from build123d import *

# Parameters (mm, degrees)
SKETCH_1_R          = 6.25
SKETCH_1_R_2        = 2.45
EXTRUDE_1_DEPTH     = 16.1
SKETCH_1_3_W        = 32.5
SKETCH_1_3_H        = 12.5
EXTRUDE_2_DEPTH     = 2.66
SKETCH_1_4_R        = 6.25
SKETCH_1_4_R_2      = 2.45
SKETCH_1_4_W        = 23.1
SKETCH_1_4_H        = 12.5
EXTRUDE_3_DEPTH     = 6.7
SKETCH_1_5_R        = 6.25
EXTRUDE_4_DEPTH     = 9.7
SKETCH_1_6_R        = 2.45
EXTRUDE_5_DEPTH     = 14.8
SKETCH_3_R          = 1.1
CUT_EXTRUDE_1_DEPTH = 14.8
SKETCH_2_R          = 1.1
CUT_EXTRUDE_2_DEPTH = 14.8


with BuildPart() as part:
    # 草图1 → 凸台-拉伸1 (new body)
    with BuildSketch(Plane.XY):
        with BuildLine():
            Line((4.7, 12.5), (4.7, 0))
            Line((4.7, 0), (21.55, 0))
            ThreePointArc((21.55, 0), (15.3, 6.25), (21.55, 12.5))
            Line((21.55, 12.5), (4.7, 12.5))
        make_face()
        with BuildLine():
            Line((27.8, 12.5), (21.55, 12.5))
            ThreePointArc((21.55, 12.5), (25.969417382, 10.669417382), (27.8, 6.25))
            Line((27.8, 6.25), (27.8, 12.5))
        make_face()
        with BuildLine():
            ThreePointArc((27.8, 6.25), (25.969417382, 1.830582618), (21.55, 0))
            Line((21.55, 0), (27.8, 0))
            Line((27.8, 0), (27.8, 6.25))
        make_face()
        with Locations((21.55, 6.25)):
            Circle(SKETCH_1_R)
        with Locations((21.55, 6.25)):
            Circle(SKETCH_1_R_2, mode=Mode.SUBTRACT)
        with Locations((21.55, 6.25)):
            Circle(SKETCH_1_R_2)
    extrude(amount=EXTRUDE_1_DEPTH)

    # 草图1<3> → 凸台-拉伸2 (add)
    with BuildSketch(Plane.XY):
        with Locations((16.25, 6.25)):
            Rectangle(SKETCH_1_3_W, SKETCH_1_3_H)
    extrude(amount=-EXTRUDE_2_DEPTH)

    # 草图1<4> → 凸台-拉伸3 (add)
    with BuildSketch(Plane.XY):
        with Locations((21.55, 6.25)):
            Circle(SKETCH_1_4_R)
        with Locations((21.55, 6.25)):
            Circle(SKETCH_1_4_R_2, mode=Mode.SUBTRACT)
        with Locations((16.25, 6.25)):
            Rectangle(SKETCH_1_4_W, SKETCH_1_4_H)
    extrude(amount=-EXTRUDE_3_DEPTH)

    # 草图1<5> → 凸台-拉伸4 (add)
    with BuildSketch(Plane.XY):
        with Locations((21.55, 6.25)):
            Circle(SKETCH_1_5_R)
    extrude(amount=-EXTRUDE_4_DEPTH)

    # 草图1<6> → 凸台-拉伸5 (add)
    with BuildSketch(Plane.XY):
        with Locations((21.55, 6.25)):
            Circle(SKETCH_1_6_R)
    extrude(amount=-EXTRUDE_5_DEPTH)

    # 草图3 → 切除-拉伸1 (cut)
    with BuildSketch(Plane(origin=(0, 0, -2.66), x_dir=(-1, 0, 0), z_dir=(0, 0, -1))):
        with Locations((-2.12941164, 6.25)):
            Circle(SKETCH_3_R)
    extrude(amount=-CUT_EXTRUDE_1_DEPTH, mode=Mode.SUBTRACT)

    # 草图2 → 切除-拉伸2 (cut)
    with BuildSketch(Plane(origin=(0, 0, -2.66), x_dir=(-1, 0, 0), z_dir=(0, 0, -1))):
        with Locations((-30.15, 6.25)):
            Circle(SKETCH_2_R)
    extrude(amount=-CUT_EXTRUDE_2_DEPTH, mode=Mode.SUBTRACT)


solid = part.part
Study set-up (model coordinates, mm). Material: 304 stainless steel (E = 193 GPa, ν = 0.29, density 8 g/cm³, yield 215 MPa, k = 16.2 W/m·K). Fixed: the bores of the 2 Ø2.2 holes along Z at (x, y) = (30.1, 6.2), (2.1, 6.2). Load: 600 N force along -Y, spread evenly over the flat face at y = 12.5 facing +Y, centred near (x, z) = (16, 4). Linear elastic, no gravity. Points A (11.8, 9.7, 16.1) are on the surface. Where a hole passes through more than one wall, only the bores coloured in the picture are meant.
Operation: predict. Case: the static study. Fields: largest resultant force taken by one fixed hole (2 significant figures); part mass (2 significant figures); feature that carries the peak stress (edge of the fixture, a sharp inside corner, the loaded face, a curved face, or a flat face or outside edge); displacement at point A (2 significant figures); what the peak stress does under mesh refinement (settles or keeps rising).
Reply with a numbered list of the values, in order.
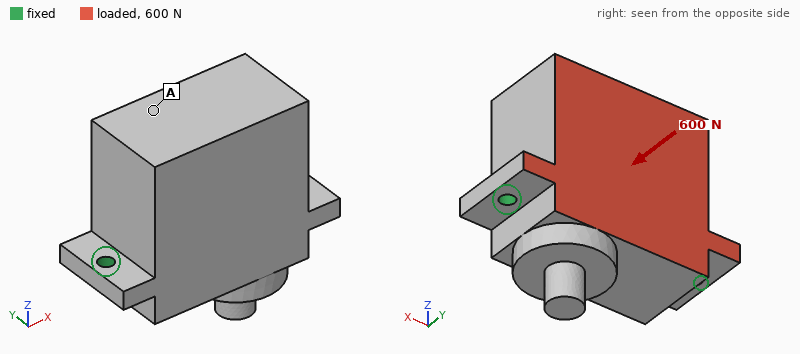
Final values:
1. 300 N
2. 59 g
3. edge of the fixture
4. 20 µm
5. keeps rising
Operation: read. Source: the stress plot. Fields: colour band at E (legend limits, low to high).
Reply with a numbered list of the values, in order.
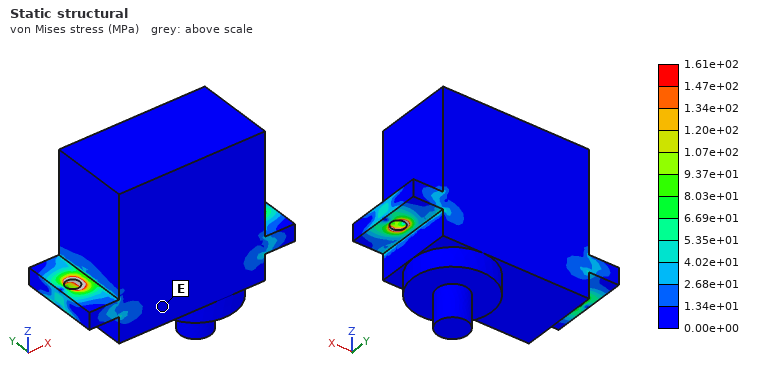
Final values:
1. 0.00e+00 to 1.34e+01 MPa
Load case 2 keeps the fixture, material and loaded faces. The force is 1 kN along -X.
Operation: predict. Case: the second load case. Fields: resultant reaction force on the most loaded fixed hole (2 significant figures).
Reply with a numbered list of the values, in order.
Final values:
1. 600 N
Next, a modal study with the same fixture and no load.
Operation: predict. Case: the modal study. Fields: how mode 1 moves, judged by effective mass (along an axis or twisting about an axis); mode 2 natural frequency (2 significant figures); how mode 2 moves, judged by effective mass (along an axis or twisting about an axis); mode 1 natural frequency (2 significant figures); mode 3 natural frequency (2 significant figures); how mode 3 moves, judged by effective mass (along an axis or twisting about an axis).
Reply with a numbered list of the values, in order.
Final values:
1. along Y
2. 15 kHz
3. along Z
4. 4000 Hz
5. 16 kHz
6. along X
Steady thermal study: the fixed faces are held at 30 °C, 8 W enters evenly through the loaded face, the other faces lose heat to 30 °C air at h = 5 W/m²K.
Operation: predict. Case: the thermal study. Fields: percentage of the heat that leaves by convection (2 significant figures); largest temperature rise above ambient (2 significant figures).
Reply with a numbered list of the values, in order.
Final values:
1. 4.8 %
2. 50 K
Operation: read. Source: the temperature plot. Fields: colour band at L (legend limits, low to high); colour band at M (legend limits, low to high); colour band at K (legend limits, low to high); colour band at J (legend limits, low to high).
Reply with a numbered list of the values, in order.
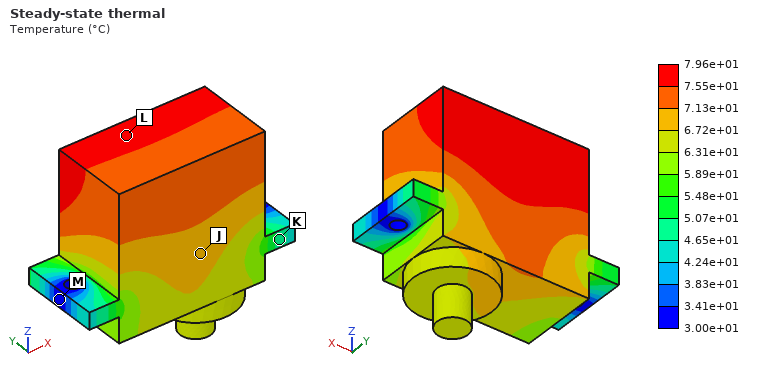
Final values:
1. 7.55e+01 to 7.96e+01 °C
2. 3.00e+01 to 3.41e+01 °C
3. 4.65e+01 to 5.07e+01 °C
4. 6.72e+01 to 7.13e+01 °C
